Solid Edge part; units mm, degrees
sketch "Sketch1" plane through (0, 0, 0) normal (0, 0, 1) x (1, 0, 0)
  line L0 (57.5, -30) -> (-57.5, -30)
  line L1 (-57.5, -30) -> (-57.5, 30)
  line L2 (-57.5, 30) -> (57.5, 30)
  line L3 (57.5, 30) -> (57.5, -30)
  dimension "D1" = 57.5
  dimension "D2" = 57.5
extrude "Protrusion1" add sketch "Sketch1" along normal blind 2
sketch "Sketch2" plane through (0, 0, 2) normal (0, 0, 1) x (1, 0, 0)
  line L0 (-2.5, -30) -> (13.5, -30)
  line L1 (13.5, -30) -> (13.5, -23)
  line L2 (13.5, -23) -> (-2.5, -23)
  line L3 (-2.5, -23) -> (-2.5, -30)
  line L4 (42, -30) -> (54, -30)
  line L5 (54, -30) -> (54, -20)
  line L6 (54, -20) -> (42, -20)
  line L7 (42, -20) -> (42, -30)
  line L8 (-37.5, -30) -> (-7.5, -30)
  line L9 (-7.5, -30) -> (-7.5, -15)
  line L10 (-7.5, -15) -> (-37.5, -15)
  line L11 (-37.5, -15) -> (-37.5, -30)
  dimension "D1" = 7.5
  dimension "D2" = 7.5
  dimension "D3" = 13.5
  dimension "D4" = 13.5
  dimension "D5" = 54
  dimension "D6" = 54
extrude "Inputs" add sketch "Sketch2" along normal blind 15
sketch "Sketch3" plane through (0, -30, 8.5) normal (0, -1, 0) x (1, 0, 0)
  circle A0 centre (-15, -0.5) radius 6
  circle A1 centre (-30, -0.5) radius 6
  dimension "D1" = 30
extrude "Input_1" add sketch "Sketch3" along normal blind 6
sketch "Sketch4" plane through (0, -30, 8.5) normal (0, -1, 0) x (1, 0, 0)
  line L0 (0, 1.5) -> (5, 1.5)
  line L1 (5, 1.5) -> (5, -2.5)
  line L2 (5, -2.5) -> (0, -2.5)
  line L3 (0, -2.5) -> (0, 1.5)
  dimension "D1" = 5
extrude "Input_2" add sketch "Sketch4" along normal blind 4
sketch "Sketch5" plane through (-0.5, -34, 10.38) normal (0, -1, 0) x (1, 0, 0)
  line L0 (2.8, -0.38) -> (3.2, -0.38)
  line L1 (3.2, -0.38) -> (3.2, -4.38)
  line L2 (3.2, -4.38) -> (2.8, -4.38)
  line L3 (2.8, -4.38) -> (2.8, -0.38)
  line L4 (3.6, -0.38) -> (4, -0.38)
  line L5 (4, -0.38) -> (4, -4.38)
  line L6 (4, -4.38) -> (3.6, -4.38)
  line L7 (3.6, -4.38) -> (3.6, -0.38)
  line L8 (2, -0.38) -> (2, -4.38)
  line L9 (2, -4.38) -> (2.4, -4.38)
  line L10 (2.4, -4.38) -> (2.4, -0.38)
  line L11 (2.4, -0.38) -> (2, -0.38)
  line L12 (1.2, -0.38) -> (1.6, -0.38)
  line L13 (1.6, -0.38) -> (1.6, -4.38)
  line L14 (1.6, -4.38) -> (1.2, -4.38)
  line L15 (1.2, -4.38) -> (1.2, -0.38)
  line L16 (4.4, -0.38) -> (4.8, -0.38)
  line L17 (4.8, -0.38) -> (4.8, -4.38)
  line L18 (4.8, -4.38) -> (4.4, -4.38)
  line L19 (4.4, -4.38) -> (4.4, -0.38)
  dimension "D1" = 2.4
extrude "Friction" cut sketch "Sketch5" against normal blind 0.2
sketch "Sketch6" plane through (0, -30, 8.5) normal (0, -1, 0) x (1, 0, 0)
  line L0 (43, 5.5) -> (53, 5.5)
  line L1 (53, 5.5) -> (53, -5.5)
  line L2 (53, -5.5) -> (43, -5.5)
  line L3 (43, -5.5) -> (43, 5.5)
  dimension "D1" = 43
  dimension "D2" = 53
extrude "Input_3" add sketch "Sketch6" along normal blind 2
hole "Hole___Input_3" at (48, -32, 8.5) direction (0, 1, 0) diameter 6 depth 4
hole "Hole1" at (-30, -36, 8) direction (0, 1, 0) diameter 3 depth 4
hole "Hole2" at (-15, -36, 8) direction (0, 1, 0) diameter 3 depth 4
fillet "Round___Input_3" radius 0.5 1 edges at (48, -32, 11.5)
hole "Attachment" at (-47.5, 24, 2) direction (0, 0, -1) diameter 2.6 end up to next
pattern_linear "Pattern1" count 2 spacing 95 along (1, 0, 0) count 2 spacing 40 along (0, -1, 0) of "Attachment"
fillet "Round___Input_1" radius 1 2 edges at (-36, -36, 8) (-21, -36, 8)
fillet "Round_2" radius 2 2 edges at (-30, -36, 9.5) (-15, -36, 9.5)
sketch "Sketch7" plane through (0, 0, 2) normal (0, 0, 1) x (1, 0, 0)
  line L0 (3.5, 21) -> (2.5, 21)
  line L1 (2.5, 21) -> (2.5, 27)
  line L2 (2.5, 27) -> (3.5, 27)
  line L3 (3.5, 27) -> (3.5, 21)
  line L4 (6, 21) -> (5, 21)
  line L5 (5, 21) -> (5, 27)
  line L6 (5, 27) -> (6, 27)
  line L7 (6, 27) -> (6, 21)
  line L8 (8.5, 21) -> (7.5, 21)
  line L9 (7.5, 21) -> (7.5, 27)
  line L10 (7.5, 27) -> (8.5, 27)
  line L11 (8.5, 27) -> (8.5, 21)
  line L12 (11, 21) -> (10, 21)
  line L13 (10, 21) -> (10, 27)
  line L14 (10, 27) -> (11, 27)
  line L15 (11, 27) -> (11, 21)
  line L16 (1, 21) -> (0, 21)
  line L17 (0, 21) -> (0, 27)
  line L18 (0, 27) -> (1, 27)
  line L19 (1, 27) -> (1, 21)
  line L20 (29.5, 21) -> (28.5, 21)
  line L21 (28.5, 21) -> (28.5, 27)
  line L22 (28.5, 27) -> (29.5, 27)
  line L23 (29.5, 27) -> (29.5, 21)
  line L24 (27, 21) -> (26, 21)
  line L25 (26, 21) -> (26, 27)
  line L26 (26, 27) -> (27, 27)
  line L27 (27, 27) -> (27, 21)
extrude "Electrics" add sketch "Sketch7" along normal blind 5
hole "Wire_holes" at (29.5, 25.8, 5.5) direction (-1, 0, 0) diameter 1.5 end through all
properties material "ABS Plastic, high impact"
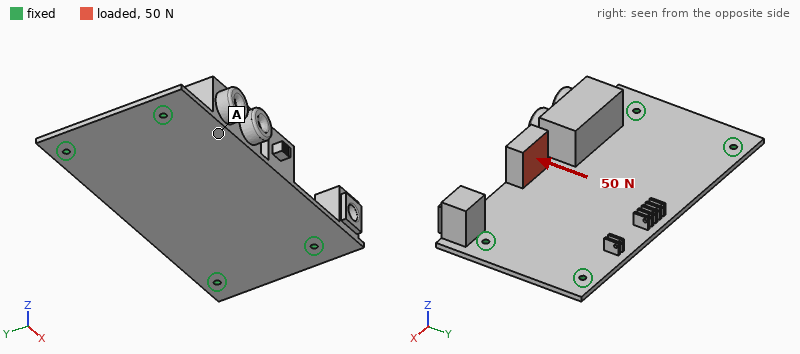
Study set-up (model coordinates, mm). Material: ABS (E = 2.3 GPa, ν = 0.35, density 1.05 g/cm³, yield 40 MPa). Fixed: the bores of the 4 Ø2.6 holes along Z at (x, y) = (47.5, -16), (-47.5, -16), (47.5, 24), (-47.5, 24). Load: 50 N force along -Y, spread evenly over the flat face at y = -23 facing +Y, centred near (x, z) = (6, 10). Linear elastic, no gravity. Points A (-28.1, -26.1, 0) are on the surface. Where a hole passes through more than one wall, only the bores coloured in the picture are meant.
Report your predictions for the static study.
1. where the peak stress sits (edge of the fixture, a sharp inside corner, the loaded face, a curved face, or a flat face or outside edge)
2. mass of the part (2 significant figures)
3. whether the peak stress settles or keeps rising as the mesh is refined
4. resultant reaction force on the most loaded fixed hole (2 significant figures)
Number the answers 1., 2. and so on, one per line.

1. edge of the fixture
2. 27 g
3. keeps rising
4. 19 N
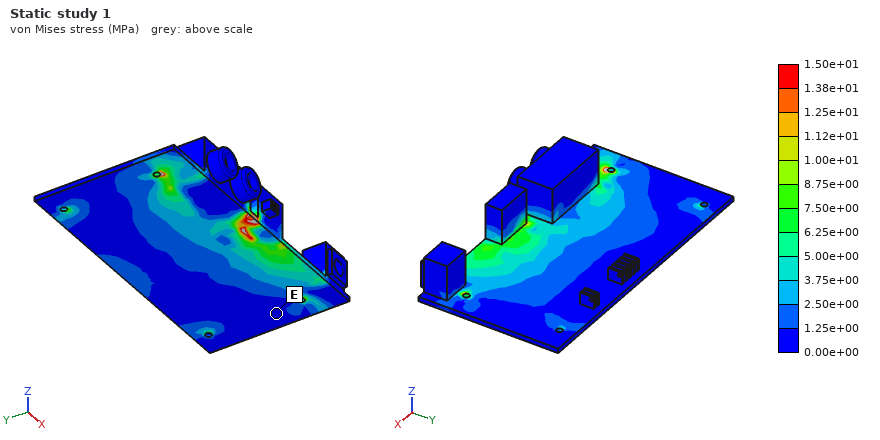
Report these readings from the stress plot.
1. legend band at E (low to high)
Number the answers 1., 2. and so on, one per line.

1. 0.00e+00 to 1.25e+00 MPa
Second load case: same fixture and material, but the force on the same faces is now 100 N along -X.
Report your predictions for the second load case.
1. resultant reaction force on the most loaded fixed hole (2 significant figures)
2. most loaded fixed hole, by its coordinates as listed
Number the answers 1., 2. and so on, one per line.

1. 48 N
2. (-47.5, -16)
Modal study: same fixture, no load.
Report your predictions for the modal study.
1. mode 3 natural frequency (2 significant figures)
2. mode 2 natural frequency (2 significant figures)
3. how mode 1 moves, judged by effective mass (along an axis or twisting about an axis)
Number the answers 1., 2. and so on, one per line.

1. 630 Hz
2. 350 Hz
3. along Z
